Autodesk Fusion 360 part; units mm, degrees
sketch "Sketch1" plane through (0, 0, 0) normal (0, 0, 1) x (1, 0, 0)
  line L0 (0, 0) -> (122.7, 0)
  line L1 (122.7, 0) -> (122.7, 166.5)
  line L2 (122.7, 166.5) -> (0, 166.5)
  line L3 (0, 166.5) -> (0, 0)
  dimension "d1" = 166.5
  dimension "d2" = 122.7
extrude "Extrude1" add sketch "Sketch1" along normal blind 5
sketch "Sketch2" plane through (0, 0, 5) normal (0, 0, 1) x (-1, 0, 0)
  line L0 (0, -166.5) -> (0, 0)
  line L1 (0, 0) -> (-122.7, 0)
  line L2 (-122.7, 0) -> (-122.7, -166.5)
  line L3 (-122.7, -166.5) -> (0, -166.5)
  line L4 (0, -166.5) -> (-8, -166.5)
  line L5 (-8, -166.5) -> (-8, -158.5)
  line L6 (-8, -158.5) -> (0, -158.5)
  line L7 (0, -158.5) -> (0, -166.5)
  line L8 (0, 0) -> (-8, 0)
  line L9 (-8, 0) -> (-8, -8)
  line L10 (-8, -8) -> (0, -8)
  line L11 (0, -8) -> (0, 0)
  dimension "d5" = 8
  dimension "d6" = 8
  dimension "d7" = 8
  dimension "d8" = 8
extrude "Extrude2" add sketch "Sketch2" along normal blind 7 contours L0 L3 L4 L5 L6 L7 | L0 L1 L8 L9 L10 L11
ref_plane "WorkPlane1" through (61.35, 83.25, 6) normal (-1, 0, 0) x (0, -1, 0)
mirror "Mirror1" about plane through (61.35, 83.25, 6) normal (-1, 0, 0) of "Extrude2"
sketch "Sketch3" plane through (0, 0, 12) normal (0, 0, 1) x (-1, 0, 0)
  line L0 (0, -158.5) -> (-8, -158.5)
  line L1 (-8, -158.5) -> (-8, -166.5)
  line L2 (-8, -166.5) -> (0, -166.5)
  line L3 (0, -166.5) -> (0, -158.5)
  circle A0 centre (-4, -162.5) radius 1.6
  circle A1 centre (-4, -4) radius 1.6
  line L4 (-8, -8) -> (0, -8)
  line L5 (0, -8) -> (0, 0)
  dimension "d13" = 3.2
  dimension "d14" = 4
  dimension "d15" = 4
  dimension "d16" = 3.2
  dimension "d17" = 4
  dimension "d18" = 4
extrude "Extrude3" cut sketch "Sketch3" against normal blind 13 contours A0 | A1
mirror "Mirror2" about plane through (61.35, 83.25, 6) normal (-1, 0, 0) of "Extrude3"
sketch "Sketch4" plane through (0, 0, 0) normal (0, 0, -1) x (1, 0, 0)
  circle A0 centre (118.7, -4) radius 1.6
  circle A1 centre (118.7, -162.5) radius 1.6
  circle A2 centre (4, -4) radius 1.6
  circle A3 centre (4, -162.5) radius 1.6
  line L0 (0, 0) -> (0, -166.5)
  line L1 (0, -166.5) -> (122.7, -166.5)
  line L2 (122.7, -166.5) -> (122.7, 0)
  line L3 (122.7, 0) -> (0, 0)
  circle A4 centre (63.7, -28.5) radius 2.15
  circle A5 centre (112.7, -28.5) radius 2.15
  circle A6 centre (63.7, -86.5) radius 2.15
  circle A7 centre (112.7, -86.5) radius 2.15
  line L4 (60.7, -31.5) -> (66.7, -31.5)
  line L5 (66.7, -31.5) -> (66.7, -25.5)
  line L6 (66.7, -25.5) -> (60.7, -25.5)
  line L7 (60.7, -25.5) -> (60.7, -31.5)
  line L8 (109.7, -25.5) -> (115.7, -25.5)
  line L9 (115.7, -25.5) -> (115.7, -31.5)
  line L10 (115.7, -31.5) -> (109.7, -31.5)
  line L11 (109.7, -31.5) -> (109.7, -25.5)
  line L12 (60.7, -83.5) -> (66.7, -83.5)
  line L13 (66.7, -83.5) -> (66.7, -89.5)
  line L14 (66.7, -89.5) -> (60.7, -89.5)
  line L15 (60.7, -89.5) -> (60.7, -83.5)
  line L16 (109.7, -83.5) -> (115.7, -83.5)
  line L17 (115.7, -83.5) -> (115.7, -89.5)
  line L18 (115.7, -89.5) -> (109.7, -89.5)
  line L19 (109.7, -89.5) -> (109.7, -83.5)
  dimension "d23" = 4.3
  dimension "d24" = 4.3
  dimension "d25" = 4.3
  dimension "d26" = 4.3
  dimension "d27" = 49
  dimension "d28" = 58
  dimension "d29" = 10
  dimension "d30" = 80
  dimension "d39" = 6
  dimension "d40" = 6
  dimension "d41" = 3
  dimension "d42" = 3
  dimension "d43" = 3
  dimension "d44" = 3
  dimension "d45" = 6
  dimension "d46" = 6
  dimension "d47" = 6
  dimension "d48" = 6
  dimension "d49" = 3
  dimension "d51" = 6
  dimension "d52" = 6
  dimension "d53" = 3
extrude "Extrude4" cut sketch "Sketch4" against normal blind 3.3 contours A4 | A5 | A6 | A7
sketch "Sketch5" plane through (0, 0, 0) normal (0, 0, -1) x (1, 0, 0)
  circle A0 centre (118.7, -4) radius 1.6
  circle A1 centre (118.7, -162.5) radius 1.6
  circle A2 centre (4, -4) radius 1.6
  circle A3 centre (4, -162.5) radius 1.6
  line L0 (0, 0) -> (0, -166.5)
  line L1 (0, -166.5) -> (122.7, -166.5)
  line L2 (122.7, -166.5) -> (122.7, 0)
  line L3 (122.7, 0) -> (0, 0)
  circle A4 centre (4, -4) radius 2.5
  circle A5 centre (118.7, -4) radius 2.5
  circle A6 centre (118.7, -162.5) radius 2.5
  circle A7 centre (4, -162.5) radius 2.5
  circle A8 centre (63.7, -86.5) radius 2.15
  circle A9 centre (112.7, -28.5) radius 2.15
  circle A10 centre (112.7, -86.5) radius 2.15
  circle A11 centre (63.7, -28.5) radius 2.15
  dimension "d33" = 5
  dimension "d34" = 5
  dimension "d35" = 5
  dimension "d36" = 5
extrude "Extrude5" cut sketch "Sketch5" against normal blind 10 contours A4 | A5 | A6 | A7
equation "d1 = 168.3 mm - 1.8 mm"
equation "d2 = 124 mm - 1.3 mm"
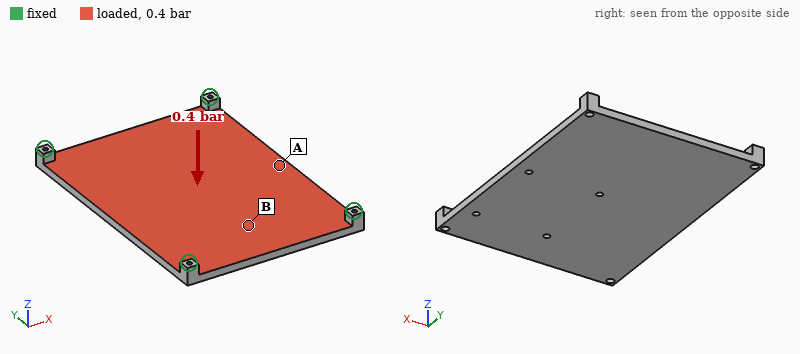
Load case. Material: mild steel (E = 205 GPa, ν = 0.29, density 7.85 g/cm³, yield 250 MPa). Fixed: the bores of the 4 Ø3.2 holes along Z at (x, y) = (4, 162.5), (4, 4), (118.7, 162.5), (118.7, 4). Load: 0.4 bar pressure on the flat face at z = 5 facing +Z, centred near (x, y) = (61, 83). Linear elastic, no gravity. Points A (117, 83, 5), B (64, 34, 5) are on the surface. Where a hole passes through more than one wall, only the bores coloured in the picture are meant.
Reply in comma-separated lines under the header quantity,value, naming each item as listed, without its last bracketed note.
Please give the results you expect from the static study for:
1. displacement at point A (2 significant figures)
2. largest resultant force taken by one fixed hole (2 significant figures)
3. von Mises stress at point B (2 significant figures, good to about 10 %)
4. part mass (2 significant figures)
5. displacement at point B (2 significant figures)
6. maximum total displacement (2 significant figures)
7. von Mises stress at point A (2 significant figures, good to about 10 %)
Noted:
quantity,value
displacement at point A,68 µm
largest resultant force taken by one fixed hole,460 N
von Mises stress at point B,8.6 MPa
part mass,810 g
displacement at point B,49 µm
maximum total displacement,77 µm
von Mises stress at point A,16 MPa
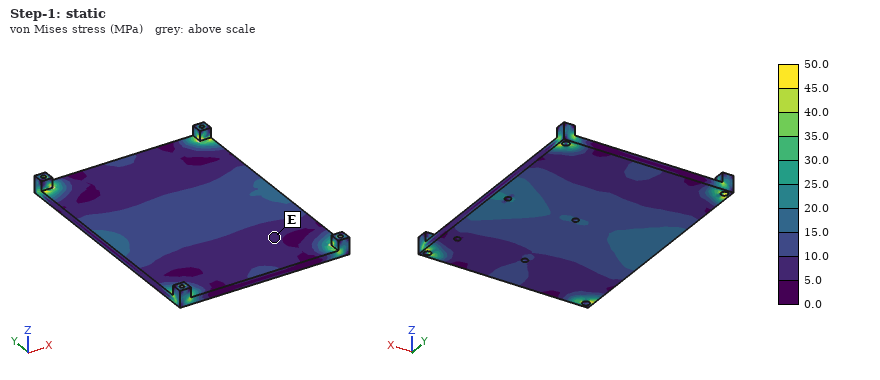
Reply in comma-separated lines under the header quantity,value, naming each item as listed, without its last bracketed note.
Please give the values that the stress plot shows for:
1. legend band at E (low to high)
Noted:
quantity,value
legend band at E,5.0 to 10.0 MPa
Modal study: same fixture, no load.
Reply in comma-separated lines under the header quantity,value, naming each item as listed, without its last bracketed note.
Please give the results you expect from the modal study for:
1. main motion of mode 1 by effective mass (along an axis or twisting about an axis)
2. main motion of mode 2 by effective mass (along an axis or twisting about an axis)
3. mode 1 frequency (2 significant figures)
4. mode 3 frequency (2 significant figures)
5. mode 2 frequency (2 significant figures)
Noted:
quantity,value
main motion of mode 1 by effective mass,along Z
main motion of mode 2 by effective mass,twisting about Y
mode 1 frequency,670 Hz
mode 3 frequency,1500 Hz
mode 2 frequency,1200 Hz
